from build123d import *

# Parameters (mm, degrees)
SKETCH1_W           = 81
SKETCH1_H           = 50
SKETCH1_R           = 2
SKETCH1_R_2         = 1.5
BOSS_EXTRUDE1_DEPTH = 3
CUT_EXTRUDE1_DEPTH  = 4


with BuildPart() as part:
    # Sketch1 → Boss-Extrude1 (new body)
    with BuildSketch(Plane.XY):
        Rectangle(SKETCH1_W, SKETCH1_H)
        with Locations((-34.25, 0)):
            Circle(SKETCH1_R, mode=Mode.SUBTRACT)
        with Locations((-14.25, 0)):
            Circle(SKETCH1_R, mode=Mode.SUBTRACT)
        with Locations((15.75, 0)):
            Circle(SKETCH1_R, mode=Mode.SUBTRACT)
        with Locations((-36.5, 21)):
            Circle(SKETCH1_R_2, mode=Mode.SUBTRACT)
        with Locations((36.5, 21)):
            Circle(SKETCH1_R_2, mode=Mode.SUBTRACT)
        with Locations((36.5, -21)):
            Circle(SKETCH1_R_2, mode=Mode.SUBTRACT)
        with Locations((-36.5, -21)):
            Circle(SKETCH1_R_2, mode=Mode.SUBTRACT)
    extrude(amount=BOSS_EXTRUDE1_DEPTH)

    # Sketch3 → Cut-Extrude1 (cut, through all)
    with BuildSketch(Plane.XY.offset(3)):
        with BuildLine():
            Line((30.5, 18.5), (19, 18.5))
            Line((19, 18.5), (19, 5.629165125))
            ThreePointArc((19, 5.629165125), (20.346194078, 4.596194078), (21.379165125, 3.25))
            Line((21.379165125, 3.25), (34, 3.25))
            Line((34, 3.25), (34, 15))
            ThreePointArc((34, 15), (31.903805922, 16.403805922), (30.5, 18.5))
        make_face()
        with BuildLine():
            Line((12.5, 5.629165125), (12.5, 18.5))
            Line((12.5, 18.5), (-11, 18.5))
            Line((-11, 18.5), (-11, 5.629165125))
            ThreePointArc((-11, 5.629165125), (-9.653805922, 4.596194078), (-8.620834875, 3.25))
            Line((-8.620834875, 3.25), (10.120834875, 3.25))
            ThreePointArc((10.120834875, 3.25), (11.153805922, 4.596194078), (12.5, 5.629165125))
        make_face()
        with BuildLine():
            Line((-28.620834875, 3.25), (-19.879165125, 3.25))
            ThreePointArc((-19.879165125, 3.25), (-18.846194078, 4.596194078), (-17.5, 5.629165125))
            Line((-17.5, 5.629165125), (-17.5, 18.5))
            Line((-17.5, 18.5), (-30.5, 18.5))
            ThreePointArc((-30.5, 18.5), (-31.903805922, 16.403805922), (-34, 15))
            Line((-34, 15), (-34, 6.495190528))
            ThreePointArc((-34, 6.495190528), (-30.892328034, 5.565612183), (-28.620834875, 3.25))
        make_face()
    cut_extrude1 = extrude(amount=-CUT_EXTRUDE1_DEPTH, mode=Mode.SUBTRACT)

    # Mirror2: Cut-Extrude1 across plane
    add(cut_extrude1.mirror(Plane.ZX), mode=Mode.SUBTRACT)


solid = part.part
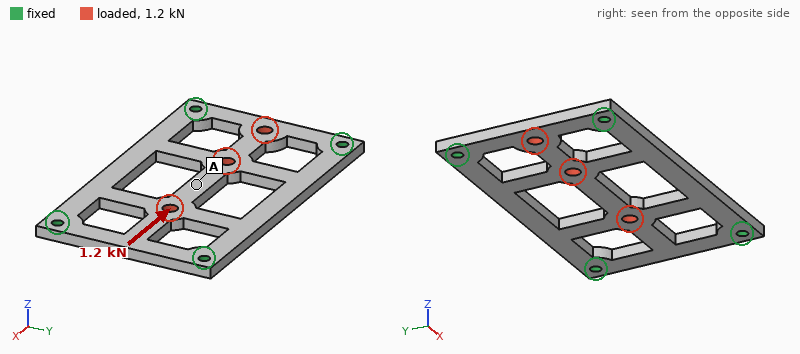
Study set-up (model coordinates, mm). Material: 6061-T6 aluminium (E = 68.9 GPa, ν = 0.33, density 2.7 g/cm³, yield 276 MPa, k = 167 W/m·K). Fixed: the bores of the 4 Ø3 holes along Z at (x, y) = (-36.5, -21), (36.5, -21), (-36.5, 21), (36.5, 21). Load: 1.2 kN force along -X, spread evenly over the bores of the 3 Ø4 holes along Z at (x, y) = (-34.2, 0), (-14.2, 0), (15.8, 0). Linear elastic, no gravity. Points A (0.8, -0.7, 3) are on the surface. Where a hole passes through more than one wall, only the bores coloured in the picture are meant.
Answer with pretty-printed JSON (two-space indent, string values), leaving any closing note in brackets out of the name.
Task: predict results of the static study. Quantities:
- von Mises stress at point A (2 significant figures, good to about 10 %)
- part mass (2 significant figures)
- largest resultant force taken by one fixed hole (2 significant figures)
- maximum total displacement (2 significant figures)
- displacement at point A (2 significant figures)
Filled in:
{
  "von Mises stress at point A": "5.2 MPa",
  "part mass": "19 g",
  "largest resultant force taken by one fixed hole": "340 N",
  "maximum total displacement": "26 µm",
  "displacement at point A": "22 µm"
}
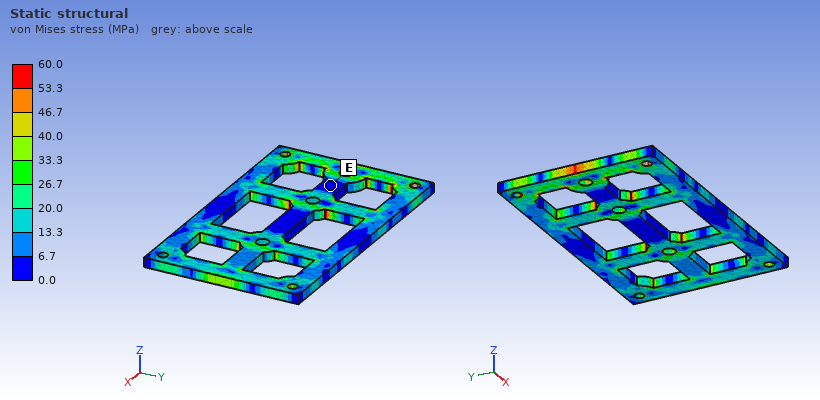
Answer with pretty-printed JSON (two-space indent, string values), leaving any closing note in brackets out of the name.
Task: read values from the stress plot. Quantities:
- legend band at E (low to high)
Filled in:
{
  "legend band at E": "0.0 to 6.7 MPa"
}
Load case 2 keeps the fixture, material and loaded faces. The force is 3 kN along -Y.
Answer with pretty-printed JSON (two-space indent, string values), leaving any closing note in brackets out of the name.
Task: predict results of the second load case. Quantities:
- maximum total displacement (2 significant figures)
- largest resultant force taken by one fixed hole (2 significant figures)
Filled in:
{
  "maximum total displacement": "71 µm",
  "largest resultant force taken by one fixed hole": "1.0 kN"
}
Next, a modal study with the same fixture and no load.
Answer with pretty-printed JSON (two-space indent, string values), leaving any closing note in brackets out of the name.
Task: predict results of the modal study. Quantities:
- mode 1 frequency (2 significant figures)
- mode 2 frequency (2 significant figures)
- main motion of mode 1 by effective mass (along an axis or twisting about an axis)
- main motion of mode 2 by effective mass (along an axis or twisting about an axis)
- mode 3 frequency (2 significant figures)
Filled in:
{
  "mode 1 frequency": "2400 Hz",
  "mode 2 frequency": "3600 Hz",
  "main motion of mode 1 by effective mass": "along Z",
  "main motion of mode 2 by effective mass": "twisting about X",
  "mode 3 frequency": "5500 Hz"
}
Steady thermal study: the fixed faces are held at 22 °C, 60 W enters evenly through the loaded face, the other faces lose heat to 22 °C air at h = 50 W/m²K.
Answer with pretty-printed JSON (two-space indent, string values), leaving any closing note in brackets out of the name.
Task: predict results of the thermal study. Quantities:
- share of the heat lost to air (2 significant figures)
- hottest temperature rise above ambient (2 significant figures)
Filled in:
{
  "share of the heat lost to air": "19 %",
  "hottest temperature rise above ambient": "75 K"
}
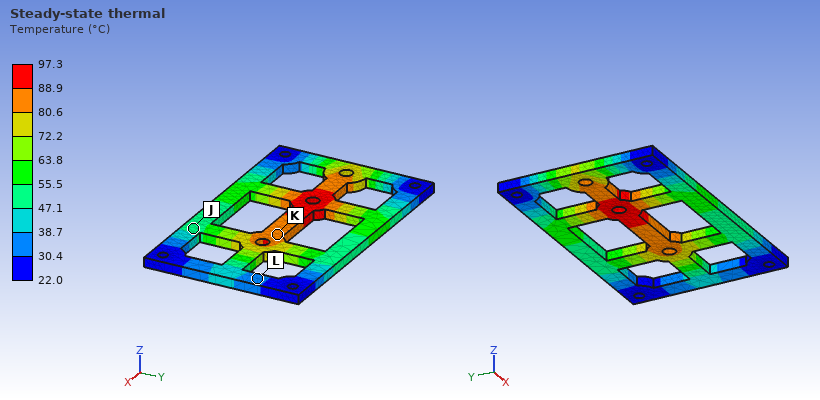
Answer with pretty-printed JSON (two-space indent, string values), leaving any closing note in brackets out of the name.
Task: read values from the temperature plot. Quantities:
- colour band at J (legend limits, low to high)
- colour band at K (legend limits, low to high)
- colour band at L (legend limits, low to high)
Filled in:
{
  "colour band at J": "47.1 to 55.5 °C",
  "colour band at K": "80.6 to 88.9 °C",
  "colour band at L": "30.4 to 38.7 °C"
}
